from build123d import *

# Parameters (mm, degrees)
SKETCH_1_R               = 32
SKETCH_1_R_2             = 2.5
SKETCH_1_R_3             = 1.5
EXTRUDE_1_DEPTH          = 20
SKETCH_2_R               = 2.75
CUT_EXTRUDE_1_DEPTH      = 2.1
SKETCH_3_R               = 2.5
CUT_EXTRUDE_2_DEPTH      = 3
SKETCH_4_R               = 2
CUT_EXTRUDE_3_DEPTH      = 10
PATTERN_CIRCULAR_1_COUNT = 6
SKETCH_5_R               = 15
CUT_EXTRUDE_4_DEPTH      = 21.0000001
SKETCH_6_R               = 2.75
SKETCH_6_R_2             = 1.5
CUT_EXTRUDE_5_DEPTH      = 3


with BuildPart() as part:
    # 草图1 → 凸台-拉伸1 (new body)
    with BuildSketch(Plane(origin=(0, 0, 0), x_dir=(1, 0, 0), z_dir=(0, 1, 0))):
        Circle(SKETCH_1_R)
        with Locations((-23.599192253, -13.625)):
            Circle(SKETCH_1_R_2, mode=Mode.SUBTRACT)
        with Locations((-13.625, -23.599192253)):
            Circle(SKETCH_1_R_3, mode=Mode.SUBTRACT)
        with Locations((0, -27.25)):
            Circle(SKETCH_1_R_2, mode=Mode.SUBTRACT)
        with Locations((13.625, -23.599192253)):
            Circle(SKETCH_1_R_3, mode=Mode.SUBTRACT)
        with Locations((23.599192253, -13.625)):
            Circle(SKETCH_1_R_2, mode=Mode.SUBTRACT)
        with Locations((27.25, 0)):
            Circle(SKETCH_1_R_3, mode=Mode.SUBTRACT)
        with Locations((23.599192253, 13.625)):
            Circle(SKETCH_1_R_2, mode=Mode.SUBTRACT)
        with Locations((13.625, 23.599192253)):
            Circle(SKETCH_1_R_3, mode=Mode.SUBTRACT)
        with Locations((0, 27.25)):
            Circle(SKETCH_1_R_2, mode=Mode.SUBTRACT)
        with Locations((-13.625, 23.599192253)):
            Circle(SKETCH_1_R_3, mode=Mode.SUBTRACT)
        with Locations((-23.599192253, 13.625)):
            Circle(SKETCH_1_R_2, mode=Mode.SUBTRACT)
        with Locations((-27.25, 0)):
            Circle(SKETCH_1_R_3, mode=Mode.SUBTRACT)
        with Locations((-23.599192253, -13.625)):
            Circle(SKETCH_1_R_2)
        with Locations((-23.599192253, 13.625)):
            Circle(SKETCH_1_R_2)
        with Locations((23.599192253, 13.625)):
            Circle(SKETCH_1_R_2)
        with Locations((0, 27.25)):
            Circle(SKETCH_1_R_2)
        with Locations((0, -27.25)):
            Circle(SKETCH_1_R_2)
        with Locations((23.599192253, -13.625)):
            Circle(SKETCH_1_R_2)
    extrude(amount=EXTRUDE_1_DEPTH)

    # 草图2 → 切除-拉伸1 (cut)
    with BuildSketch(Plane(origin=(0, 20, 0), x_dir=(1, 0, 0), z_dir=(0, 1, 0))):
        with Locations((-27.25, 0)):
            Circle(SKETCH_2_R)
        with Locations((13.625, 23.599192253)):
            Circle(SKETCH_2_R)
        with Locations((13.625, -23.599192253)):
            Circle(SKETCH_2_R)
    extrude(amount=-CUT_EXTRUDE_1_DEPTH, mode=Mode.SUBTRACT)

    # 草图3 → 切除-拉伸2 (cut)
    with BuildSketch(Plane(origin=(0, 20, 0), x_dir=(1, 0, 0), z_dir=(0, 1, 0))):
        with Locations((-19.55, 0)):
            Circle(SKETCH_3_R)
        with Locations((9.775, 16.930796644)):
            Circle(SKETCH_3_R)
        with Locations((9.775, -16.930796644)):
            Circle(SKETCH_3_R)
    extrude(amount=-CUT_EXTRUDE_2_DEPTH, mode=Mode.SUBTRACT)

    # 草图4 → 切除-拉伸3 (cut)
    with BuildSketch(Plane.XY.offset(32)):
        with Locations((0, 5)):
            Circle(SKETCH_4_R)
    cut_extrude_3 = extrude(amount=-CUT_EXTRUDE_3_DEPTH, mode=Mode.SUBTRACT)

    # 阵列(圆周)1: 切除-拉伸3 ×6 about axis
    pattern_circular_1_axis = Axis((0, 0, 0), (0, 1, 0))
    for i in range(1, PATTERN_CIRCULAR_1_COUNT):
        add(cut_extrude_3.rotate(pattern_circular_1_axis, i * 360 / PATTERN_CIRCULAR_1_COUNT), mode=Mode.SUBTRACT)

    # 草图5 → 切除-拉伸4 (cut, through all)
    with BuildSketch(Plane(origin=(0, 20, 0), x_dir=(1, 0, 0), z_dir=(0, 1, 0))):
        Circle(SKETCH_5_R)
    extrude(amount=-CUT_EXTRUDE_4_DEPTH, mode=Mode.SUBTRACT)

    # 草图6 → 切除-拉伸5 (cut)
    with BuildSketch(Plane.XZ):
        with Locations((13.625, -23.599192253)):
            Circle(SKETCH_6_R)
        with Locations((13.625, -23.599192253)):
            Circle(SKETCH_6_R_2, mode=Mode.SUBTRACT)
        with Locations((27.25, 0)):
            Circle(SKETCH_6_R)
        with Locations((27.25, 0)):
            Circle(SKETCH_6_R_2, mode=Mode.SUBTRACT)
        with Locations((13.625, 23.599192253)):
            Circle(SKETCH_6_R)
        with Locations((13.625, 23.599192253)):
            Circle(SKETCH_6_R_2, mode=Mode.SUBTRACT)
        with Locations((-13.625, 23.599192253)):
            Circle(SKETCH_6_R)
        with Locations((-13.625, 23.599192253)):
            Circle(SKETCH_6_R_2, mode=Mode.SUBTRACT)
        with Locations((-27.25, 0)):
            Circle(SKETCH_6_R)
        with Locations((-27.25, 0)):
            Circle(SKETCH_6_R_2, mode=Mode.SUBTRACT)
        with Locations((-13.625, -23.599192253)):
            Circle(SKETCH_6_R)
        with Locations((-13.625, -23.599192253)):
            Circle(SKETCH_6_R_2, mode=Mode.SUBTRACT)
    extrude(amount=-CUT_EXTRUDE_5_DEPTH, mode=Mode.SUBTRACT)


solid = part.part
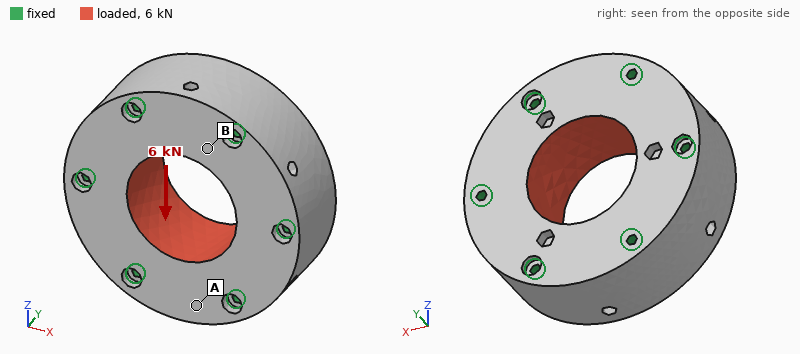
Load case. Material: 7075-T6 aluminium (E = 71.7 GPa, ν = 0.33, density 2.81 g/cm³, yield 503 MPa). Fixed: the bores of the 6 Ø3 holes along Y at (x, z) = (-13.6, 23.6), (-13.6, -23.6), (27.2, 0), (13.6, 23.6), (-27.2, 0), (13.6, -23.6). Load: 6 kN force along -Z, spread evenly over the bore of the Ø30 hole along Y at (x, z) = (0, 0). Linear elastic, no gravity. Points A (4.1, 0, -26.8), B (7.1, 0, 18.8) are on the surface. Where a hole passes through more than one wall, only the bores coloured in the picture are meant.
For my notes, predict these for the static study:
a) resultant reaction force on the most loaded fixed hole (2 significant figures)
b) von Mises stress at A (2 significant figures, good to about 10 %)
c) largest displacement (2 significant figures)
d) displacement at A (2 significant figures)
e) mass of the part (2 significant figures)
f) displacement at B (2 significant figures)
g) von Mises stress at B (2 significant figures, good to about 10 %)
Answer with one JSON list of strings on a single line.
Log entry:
["1.2 kN", "1.9 MPa", "1.5 µm", "1.1 µm", "130 g", "1.0 µm", "3.4 MPa"]
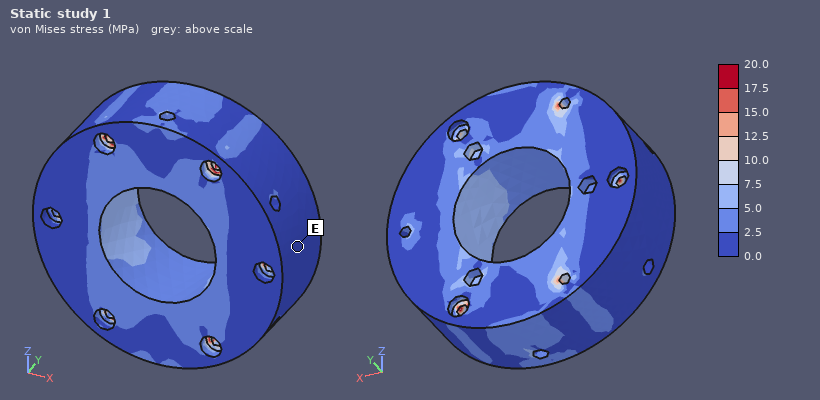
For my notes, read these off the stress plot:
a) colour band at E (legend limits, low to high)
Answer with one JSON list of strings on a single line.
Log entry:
["0.0 to 2.5 MPa"]
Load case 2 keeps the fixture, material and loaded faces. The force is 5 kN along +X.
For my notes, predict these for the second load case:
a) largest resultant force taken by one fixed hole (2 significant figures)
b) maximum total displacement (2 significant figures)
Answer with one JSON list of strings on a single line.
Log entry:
["1.1 kN", "1.2 µm"]
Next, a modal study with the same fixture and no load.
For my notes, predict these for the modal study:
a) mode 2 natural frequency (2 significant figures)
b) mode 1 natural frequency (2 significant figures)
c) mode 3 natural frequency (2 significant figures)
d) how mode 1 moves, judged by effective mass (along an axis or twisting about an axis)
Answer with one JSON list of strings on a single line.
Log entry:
["39 kHz", "34 kHz", "40 kHz", "along Y"]
